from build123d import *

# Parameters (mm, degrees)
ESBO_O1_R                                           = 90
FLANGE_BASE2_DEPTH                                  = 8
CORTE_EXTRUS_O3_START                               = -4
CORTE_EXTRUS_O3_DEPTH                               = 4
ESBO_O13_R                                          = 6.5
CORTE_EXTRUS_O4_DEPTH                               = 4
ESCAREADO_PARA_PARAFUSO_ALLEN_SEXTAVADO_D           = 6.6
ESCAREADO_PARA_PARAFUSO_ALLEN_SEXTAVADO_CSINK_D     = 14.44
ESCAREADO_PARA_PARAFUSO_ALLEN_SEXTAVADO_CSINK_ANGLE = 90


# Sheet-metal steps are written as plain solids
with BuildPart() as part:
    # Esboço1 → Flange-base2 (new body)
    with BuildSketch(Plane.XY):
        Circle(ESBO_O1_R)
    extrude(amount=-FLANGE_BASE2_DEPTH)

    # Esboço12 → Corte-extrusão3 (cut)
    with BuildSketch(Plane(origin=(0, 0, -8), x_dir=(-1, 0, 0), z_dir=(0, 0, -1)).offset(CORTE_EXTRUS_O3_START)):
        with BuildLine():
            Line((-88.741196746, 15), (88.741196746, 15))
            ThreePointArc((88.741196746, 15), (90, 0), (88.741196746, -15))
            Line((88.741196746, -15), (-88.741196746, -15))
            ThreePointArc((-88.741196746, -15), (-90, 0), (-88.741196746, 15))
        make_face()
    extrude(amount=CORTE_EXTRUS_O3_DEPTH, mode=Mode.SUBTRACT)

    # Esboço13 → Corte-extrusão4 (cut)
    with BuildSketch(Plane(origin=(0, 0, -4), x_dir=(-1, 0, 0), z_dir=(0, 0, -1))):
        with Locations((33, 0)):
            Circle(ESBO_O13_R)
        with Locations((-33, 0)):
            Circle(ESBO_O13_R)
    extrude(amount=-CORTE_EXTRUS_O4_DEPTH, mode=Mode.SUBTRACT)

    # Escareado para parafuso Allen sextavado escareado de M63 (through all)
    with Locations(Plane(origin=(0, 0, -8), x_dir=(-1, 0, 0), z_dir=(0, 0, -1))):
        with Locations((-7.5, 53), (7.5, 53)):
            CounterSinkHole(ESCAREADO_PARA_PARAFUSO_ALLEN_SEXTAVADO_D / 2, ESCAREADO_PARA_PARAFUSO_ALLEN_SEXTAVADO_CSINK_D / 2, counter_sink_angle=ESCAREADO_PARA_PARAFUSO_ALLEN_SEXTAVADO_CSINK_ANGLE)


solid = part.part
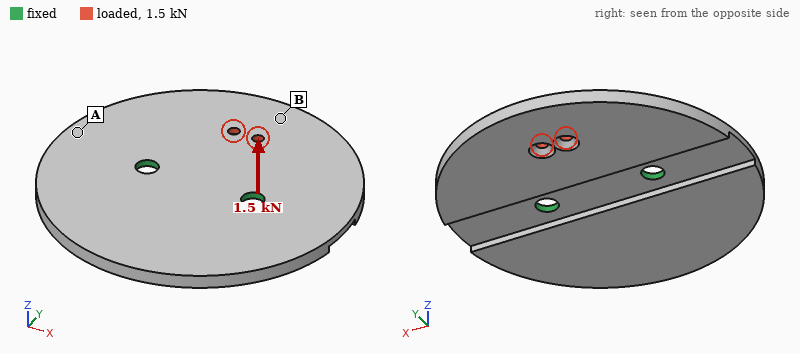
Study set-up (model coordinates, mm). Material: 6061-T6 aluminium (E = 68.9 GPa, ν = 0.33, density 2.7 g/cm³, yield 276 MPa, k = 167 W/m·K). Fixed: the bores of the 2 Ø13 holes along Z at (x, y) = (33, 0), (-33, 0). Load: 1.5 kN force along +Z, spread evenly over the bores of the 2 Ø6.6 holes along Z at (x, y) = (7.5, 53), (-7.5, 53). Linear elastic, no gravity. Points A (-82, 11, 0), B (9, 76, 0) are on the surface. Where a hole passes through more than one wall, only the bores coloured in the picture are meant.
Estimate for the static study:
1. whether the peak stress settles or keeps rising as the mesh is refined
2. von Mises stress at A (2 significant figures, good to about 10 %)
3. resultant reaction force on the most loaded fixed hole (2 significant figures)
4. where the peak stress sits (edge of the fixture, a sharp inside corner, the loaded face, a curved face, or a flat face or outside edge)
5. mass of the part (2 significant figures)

keeps rising
66 MPa
790 N
edge of the fixture
490 g
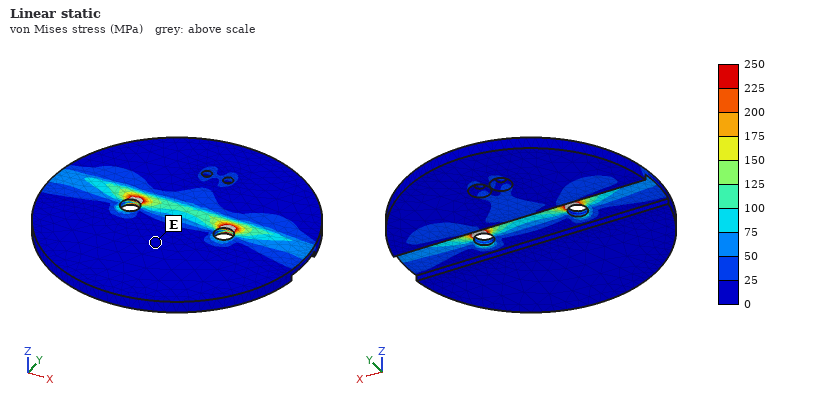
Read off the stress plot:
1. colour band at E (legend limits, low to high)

0 to 25 MPa
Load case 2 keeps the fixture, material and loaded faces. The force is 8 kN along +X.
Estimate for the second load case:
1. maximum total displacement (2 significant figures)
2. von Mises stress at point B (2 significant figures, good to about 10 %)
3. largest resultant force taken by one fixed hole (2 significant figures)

0.10 mm
8.3 MPa
7.0 kN
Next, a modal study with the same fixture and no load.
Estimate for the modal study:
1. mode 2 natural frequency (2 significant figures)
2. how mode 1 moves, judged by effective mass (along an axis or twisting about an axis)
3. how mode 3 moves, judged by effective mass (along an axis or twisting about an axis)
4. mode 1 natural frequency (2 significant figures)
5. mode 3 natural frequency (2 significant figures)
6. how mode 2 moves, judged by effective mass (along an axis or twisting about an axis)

540 Hz
twisting about X
twisting about Y
460 Hz
1100 Hz
along Z
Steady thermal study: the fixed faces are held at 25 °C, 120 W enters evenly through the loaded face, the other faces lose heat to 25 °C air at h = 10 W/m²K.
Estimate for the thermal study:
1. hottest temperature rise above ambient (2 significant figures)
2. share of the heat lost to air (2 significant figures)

74 K
9.9 %
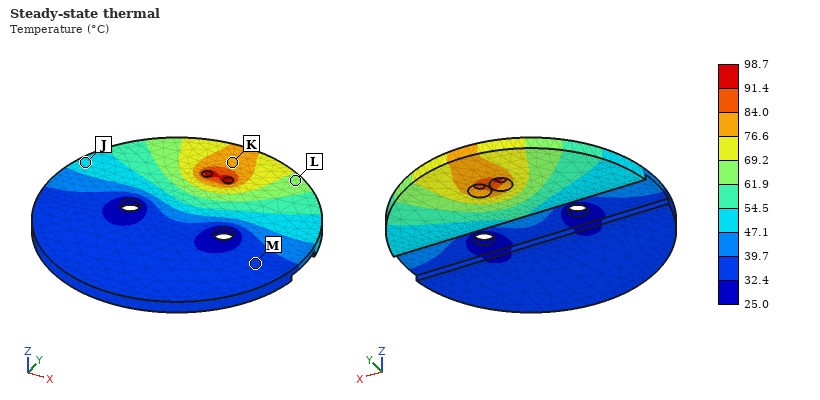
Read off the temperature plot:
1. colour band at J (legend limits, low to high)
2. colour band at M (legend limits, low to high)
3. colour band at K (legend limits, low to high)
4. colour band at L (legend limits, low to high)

47.1 to 54.5 °C
32.4 to 39.7 °C
76.6 to 84.0 °C
61.9 to 69.2 °C
